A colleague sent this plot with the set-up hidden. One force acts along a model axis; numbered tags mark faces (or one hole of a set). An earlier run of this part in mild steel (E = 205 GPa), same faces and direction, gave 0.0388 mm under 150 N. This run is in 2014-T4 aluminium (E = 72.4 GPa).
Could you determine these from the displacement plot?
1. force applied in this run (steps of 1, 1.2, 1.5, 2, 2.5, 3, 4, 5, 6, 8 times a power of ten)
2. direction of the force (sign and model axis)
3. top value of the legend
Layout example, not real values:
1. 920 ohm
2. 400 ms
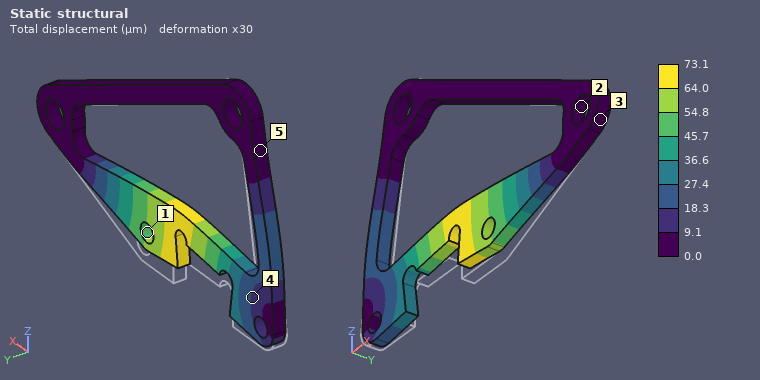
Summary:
1. 100 N
2. +Z
3. 73.1 µm
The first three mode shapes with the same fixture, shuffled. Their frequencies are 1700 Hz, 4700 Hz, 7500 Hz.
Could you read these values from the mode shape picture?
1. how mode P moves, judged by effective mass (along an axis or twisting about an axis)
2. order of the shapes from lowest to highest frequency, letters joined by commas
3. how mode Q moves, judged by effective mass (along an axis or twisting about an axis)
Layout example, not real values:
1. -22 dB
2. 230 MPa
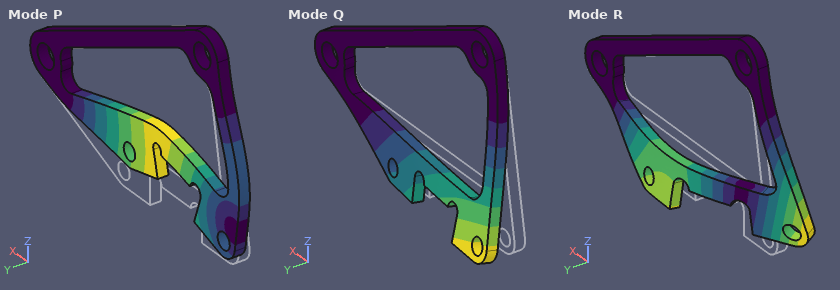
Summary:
1. along Z
2. Q, R, P
3. along Y
